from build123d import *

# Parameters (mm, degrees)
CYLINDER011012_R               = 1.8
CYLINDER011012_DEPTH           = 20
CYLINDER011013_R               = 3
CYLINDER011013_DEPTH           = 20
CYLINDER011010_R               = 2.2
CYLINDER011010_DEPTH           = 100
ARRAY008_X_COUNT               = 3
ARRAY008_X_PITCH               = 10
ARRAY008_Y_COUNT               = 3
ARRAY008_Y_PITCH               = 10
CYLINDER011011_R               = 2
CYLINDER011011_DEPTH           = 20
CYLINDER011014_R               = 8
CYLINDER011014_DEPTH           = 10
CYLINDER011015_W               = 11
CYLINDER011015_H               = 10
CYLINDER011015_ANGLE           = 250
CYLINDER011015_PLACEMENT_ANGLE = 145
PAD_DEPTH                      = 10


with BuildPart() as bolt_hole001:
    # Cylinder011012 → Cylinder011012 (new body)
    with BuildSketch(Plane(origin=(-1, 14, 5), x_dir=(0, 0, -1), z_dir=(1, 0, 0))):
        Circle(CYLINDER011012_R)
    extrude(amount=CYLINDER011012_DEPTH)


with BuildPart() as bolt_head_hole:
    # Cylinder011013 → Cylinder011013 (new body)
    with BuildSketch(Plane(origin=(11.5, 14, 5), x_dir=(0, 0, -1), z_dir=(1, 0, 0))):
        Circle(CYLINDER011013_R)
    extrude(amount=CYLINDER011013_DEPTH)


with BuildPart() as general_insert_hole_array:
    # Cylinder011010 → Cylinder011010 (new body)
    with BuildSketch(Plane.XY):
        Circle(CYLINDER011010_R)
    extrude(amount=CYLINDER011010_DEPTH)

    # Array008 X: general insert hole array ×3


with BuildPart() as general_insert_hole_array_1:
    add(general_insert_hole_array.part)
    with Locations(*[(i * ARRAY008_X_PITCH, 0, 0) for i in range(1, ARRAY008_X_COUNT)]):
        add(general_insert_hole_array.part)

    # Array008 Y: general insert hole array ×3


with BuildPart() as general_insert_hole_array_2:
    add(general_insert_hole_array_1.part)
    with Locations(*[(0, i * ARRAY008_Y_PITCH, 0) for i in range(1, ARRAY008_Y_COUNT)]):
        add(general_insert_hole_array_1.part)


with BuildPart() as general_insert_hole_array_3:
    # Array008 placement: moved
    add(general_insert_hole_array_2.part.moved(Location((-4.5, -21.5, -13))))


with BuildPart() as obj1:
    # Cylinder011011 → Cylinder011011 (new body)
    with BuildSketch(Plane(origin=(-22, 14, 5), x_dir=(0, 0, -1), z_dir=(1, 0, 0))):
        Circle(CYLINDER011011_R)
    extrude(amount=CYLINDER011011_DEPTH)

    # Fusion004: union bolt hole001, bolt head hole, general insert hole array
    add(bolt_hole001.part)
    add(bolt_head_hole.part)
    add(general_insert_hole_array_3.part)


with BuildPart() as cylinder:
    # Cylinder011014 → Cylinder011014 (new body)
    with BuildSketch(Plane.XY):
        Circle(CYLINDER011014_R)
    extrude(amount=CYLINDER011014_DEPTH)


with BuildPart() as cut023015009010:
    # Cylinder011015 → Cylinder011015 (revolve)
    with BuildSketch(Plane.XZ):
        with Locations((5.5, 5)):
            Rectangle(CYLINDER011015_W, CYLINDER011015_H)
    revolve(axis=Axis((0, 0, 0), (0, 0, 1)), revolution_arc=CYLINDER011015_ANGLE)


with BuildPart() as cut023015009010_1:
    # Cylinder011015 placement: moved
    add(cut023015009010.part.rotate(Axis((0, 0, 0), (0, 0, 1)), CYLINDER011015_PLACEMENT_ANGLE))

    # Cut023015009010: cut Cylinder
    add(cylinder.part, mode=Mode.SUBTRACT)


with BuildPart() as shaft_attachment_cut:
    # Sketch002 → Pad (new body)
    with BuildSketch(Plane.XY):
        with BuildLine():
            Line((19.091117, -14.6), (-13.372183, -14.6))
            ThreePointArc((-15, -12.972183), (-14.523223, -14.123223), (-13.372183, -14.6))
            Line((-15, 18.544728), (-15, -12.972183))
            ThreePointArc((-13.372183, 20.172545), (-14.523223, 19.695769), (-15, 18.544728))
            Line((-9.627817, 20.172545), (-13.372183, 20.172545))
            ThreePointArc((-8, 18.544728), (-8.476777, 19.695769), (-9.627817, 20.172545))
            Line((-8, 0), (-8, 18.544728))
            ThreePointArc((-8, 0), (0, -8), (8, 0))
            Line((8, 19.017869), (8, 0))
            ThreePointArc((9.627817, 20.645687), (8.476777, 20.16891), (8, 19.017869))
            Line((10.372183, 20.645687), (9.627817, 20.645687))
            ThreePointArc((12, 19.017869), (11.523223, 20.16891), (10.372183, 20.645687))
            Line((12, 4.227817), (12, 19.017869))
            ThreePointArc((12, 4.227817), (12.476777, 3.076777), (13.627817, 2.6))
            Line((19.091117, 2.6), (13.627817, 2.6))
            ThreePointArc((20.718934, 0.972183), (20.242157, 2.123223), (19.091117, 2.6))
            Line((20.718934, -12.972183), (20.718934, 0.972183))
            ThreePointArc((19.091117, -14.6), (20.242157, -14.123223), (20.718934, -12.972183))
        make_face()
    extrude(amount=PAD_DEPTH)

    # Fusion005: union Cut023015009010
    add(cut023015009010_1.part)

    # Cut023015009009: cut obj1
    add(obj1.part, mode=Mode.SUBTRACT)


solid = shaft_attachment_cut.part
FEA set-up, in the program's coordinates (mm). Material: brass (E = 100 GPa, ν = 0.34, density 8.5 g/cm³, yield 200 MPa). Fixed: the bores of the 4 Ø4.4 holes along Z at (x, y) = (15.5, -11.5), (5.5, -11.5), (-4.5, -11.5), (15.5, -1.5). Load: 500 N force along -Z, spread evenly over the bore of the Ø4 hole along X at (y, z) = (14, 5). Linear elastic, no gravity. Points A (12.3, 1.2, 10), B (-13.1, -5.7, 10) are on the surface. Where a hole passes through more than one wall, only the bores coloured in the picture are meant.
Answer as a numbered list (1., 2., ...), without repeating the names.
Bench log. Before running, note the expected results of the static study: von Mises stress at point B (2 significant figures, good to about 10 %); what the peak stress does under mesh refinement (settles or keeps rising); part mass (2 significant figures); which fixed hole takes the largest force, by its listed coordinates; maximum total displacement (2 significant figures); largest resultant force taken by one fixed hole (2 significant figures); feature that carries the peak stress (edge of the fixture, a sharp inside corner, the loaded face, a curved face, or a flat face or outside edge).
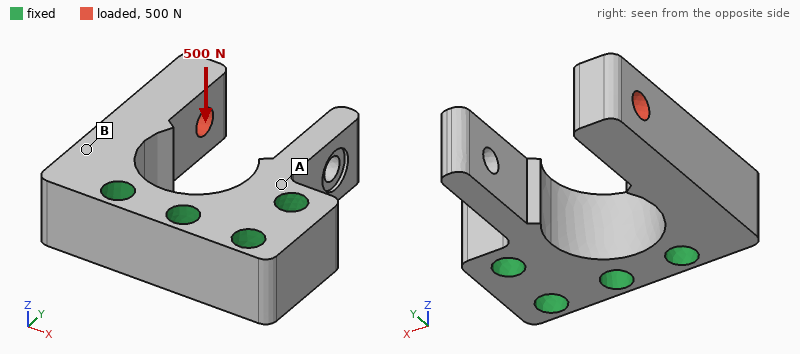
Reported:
1. 56 MPa
2. keeps rising
3. 51 g
4. (-4.5, -11.5)
5. 77 µm
6. 510 N
7. edge of the fixture
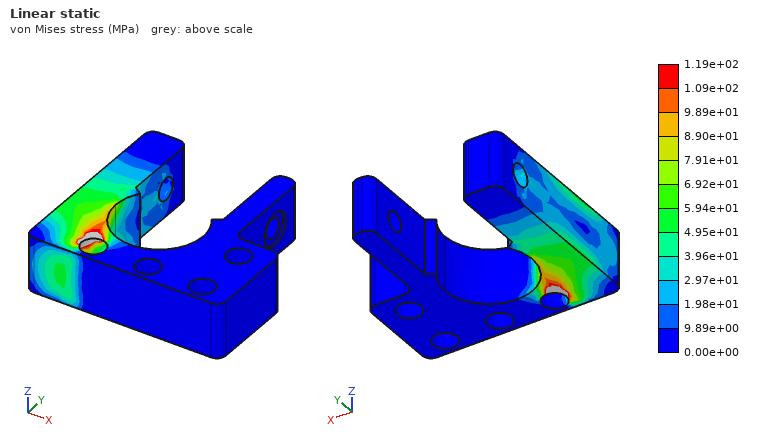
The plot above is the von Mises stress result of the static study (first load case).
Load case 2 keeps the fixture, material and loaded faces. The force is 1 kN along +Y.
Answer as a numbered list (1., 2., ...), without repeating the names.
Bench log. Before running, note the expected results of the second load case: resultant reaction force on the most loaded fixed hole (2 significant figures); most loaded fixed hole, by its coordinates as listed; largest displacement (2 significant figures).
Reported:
1. 1.1 kN
2. (-4.5, -11.5)
3. 24 µm
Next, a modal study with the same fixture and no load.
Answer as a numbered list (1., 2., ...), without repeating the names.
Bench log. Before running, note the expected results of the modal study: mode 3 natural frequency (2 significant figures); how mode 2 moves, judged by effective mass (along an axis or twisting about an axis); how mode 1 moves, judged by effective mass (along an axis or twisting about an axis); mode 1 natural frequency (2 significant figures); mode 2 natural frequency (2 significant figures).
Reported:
1. 6300 Hz
2. along Z
3. along X
4. 4300 Hz
5. 5200 Hz
